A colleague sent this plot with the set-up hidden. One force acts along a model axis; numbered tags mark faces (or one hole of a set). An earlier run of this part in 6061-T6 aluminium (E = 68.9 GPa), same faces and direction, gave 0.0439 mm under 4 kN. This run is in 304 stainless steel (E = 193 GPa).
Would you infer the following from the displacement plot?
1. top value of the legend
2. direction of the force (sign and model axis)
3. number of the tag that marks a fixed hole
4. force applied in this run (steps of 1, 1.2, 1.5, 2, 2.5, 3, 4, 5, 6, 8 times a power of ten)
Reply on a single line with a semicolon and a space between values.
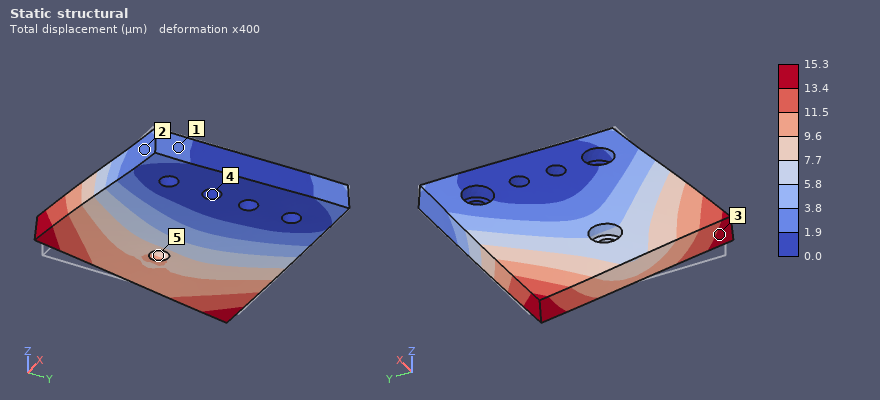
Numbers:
15.3 µm; -Y; 4; 4 kN
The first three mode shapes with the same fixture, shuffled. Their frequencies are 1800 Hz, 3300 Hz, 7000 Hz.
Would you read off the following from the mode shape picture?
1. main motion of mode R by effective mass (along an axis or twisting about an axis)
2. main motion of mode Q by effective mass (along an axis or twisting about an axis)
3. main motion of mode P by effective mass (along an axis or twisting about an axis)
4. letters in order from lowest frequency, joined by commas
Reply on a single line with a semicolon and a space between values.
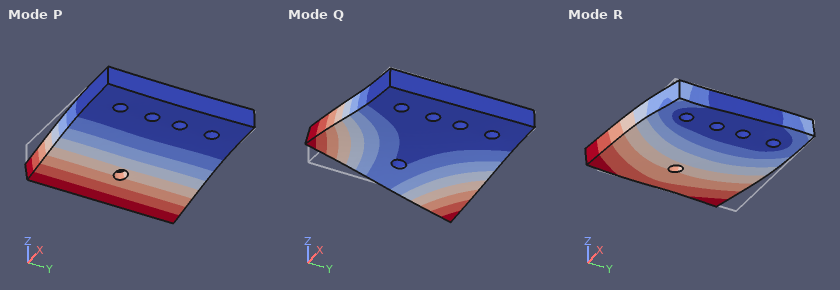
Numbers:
along Y; twisting about X; along Z; P, Q, R
